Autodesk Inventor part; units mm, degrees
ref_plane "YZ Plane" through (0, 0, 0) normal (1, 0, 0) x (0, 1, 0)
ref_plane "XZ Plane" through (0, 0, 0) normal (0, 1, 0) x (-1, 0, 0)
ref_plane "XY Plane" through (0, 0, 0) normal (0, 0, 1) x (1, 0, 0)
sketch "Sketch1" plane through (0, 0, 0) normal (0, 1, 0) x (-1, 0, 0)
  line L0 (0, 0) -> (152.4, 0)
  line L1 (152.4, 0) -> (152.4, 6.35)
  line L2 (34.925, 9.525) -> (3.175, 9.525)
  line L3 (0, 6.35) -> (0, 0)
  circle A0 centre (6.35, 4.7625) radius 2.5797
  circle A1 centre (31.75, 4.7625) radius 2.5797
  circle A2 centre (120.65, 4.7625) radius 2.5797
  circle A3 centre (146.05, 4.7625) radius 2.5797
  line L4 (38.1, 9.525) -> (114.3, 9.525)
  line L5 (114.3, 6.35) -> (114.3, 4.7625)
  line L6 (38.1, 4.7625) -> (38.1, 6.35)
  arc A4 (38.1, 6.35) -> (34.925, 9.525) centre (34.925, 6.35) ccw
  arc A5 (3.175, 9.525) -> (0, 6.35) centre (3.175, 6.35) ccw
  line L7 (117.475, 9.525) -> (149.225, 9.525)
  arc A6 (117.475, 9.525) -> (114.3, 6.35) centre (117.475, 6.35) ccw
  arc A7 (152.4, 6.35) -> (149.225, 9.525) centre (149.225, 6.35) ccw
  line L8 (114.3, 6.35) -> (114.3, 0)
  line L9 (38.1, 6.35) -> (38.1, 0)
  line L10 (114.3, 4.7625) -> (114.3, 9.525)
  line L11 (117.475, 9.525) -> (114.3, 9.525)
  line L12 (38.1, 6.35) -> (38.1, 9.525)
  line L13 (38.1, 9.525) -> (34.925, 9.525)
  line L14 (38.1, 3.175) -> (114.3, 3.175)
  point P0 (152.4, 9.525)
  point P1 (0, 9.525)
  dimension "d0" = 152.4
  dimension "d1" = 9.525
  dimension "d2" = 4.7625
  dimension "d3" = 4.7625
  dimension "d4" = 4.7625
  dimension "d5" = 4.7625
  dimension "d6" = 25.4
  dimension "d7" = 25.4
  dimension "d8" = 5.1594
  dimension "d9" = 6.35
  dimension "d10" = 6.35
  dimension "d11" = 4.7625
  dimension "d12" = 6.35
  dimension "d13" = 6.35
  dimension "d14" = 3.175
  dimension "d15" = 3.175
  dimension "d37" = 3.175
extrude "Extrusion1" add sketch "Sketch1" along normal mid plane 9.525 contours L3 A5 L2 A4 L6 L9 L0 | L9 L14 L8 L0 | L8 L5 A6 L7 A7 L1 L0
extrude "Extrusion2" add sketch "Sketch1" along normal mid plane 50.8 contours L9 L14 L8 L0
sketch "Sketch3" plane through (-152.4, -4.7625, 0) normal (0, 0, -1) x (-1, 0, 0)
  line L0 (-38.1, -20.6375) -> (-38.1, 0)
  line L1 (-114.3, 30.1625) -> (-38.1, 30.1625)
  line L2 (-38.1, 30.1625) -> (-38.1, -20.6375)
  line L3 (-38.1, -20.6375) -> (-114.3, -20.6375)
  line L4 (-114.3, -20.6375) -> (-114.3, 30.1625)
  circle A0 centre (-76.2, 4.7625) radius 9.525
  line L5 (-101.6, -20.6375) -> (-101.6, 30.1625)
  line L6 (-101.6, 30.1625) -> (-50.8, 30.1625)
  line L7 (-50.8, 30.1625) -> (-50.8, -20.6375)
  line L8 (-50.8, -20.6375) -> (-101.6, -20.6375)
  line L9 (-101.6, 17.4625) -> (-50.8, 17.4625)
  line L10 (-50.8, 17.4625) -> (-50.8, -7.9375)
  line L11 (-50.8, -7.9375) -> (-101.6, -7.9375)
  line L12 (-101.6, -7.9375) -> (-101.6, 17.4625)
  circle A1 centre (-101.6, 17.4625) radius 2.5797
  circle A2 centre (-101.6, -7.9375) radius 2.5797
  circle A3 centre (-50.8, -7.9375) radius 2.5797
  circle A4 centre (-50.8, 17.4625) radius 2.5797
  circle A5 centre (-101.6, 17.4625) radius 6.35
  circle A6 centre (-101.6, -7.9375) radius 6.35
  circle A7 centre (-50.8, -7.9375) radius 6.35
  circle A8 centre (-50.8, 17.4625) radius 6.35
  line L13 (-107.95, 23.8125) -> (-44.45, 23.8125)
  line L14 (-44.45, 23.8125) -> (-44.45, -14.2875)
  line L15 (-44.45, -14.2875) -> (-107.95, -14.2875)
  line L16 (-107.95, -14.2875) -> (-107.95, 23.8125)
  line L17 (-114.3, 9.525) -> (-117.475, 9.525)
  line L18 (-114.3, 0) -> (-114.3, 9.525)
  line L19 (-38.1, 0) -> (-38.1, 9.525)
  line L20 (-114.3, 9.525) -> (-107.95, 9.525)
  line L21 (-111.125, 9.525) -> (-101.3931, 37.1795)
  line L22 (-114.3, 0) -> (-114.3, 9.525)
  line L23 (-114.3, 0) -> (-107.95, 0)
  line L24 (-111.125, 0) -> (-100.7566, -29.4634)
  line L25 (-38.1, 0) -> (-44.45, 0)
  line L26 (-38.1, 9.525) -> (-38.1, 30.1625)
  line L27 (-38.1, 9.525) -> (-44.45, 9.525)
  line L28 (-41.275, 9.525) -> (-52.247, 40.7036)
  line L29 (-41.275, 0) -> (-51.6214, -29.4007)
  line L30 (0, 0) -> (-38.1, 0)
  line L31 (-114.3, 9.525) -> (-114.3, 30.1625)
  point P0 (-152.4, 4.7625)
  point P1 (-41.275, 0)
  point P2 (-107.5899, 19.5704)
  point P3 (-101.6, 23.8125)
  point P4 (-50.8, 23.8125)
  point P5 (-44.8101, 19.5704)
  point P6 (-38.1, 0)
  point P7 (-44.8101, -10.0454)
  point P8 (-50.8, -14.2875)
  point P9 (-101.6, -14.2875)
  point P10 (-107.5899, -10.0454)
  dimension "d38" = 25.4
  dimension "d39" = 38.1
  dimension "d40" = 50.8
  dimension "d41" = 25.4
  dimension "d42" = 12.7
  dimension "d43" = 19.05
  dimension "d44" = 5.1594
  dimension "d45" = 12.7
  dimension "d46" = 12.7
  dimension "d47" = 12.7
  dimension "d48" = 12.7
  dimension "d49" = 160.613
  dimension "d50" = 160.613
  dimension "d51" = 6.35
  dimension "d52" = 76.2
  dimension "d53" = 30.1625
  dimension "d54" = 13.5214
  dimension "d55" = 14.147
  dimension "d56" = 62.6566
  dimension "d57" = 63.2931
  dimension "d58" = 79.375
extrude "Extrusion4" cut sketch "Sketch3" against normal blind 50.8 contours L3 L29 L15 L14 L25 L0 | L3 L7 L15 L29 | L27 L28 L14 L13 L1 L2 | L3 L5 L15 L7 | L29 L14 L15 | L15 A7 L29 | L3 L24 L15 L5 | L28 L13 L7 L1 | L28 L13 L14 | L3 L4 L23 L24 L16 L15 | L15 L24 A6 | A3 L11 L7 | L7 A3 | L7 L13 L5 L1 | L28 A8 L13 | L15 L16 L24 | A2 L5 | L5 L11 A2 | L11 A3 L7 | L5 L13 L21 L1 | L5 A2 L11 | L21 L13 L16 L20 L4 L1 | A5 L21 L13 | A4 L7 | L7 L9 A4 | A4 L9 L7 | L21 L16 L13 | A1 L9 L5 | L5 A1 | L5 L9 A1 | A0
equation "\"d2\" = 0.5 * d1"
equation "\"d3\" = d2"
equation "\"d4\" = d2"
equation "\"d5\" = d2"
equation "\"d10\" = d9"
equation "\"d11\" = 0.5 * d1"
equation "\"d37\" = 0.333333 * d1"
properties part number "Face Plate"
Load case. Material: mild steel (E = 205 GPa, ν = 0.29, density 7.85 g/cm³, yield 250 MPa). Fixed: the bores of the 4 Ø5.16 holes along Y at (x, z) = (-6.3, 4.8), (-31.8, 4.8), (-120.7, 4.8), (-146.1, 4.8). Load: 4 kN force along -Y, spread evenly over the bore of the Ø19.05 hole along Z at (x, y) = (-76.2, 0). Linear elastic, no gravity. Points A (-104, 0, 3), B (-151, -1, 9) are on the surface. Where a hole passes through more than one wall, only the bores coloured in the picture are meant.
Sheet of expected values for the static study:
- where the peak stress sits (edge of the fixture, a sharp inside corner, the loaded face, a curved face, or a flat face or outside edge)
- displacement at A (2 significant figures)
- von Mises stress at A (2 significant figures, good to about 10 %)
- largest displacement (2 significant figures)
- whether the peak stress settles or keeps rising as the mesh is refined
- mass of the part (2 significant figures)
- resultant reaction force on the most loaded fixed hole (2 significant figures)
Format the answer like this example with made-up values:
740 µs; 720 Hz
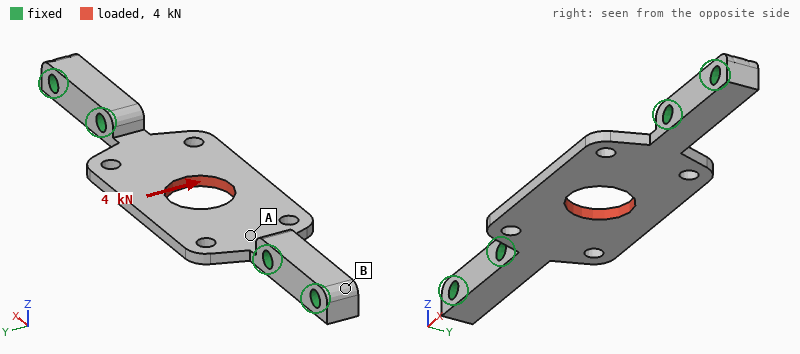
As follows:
edge of the fixture; 17 µm; 35 MPa; 30 µm; keeps rising; 100 g; 2.0 kN
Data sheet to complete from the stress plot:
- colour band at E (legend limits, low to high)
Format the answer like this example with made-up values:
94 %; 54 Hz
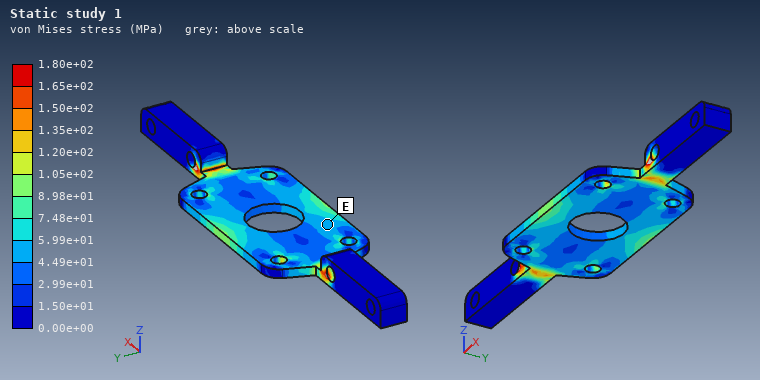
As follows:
4.49e+01 to 5.99e+01 MPa
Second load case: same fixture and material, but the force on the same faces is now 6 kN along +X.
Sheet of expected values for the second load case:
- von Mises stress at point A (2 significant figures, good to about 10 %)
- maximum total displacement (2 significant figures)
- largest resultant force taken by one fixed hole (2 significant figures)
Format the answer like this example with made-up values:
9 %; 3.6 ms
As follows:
71 MPa; 12 µm; 3.0 kN
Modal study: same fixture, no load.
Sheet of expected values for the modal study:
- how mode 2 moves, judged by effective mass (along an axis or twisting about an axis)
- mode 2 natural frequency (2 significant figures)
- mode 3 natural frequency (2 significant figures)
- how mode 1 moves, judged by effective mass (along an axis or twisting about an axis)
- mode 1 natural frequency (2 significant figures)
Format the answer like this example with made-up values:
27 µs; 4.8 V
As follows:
twisting about X; 2300 Hz; 5200 Hz; along Z; 1900 Hz
